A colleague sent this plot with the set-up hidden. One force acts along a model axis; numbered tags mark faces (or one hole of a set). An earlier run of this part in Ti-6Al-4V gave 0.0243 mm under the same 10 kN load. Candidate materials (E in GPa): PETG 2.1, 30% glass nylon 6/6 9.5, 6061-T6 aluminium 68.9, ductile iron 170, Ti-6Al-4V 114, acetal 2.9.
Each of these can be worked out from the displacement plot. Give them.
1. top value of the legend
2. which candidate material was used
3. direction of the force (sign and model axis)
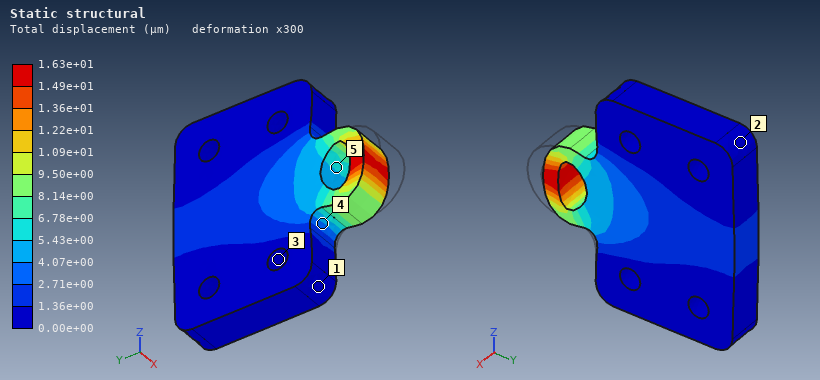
1.63e+01 µm
ductile iron
+Y
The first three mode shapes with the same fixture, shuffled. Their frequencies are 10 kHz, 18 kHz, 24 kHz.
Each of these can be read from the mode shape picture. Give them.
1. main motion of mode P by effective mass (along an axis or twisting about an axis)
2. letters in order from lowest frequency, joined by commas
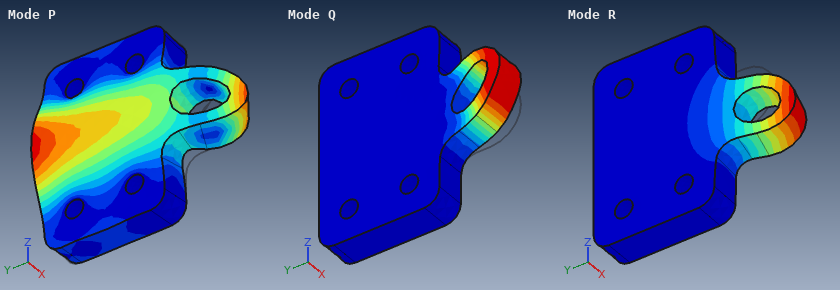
along X
R, Q, P
